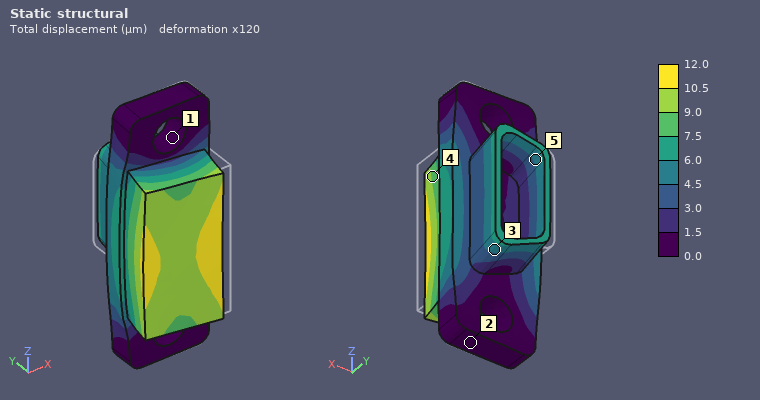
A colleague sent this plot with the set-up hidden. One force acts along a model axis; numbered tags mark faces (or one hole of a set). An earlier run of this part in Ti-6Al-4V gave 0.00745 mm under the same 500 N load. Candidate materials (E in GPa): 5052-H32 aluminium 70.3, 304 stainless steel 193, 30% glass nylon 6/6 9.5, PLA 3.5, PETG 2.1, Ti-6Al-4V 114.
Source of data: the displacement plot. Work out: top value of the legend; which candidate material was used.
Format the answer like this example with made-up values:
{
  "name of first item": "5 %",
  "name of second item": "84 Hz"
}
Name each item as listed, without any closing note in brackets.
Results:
{
  "top value of the legend": "12.0 µm",
  "which candidate material was used": "5052-H32 aluminium"
}
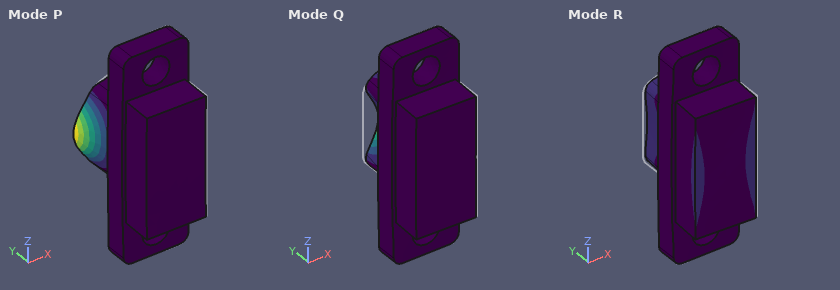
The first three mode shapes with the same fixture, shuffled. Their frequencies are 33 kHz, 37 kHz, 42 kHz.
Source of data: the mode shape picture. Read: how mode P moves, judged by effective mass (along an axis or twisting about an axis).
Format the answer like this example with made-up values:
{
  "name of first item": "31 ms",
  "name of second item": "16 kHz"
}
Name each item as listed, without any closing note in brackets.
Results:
{
  "how mode P moves, judged by effective mass": "along X"
}
